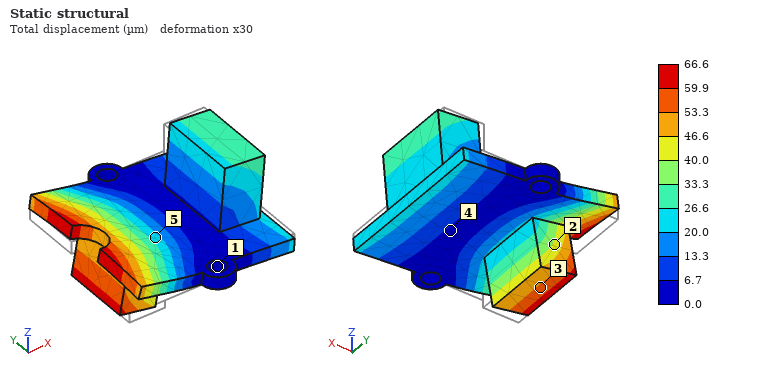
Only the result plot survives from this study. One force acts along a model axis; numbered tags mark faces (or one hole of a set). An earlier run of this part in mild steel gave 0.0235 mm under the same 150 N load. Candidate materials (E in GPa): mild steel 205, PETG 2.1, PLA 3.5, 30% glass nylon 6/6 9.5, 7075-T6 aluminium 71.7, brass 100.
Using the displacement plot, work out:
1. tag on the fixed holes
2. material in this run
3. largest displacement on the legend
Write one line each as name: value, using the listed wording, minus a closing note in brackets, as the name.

tag on the fixed holes: 1
material in this run: 7075-T6 aluminium
largest displacement on the legend: 66.6 µm
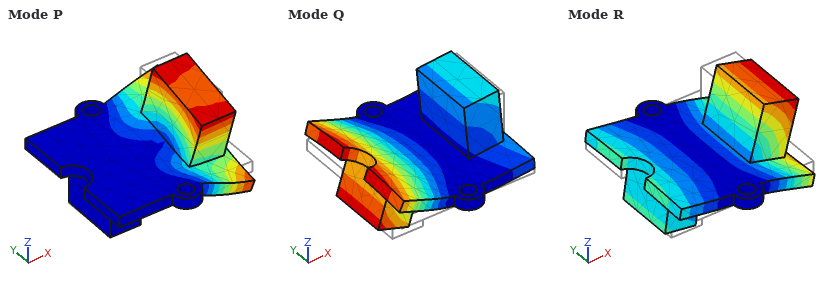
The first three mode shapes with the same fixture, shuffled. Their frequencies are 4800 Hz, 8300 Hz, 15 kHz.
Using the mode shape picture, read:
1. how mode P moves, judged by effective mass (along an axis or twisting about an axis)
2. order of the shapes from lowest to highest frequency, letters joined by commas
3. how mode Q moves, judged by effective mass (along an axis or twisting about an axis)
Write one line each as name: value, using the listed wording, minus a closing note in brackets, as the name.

how mode P moves, judged by effective mass: along Y
order of the shapes from lowest to highest frequency, letters joined by commas: R, Q, P
how mode Q moves, judged by effective mass: along Z
